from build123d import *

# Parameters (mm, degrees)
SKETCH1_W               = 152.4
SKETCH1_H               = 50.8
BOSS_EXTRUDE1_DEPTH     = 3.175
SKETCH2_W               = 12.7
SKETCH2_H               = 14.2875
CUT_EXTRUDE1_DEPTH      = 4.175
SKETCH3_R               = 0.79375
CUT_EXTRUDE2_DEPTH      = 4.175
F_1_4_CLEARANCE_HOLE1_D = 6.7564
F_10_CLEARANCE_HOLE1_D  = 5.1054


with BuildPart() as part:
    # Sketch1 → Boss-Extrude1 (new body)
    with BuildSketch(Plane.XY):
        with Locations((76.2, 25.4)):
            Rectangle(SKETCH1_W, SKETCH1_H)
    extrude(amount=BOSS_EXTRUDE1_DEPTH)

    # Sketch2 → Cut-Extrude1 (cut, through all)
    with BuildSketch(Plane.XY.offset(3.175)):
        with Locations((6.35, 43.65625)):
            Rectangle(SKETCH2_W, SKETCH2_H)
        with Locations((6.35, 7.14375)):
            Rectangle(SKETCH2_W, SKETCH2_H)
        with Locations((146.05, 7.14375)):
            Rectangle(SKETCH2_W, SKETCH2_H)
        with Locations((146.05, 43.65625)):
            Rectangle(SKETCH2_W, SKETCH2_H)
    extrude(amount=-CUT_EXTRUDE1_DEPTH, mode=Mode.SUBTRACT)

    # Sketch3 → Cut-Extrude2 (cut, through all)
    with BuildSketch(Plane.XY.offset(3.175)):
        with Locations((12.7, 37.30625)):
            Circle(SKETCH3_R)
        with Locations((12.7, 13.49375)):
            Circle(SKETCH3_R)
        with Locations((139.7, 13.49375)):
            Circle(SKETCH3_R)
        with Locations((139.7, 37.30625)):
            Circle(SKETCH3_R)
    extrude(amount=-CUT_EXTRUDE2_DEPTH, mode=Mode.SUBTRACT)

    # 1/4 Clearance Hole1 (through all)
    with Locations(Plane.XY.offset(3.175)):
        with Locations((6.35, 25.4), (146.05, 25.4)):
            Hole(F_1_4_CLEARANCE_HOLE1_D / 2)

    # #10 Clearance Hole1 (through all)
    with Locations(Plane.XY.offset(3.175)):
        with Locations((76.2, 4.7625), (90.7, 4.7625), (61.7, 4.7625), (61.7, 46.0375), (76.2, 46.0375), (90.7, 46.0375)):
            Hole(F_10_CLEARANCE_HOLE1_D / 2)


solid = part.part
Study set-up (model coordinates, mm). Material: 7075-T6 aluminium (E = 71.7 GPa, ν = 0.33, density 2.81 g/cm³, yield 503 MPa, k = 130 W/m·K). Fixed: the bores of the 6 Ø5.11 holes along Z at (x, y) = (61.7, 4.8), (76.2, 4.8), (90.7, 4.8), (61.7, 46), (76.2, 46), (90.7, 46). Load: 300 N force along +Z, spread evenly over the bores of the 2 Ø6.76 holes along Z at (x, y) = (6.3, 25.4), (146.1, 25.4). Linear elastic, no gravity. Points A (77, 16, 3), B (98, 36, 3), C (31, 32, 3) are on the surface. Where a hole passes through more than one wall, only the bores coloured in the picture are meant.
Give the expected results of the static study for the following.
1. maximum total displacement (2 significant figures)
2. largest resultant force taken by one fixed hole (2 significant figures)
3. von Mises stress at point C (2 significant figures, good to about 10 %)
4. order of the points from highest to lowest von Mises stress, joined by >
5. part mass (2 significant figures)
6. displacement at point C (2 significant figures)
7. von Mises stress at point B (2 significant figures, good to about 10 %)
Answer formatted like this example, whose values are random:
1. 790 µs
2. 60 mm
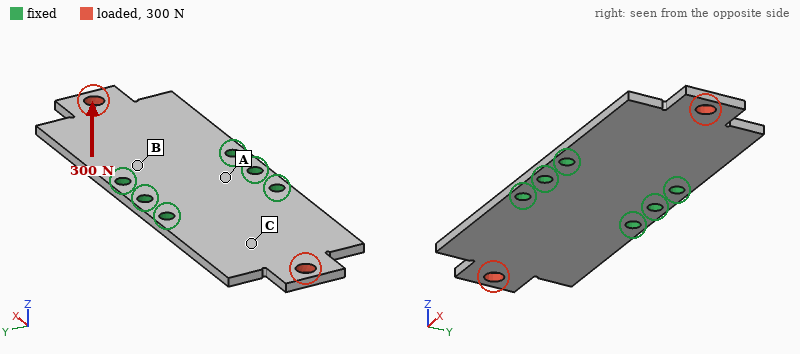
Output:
1. 1.1 mm
2. 170 N
3. 46 MPa
4. B > C > A
5. 61 g
6. 0.36 mm
7. 73 MPa
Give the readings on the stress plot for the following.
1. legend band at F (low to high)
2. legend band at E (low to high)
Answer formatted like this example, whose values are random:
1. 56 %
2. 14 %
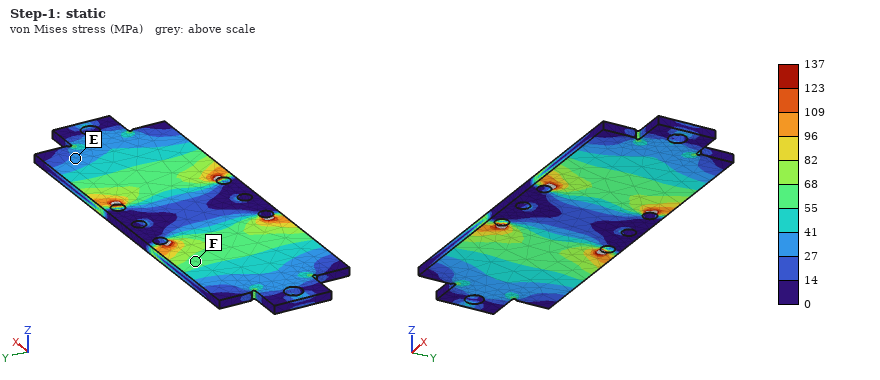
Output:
1. 55 to 68 MPa
2. 27 to 41 MPa
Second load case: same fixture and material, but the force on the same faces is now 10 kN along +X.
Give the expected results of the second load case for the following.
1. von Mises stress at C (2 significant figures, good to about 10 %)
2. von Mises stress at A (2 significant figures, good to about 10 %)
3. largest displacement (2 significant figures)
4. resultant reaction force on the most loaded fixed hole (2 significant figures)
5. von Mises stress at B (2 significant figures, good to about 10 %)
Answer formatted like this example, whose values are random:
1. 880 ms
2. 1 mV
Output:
1. 45 MPa
2. 16 MPa
3. 57 µm
4. 2.1 kN
5. 29 MPa
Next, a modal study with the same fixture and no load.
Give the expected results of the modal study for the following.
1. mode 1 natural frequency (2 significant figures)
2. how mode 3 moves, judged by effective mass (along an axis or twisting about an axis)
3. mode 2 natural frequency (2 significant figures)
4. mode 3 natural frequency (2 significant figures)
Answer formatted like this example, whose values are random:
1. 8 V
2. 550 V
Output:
1. 850 Hz
2. twisting about X
3. 850 Hz
4. 2600 Hz
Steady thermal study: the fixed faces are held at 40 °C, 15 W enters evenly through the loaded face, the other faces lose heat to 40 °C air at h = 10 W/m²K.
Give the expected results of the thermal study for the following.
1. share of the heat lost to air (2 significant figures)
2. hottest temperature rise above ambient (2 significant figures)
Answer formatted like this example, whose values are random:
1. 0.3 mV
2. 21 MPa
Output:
1. 9.0 %
2. 30 K
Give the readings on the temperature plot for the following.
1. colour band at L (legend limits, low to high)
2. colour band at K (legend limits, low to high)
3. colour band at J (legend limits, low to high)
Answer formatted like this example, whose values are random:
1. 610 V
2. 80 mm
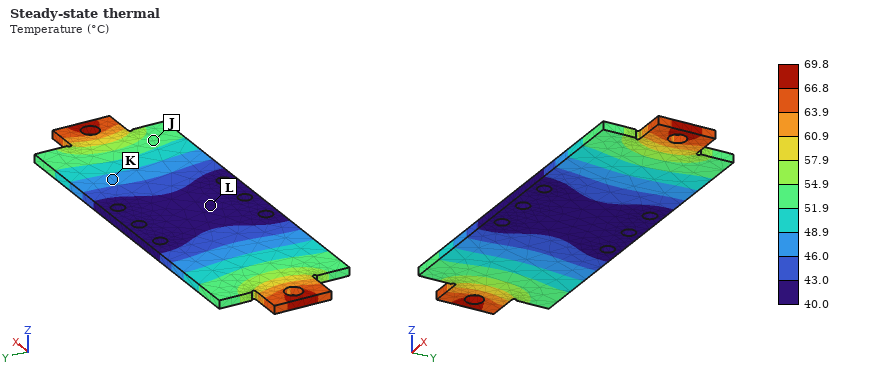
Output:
1. 40.0 to 43.0 °C
2. 46.0 to 48.9 °C
3. 51.9 to 54.9 °C
